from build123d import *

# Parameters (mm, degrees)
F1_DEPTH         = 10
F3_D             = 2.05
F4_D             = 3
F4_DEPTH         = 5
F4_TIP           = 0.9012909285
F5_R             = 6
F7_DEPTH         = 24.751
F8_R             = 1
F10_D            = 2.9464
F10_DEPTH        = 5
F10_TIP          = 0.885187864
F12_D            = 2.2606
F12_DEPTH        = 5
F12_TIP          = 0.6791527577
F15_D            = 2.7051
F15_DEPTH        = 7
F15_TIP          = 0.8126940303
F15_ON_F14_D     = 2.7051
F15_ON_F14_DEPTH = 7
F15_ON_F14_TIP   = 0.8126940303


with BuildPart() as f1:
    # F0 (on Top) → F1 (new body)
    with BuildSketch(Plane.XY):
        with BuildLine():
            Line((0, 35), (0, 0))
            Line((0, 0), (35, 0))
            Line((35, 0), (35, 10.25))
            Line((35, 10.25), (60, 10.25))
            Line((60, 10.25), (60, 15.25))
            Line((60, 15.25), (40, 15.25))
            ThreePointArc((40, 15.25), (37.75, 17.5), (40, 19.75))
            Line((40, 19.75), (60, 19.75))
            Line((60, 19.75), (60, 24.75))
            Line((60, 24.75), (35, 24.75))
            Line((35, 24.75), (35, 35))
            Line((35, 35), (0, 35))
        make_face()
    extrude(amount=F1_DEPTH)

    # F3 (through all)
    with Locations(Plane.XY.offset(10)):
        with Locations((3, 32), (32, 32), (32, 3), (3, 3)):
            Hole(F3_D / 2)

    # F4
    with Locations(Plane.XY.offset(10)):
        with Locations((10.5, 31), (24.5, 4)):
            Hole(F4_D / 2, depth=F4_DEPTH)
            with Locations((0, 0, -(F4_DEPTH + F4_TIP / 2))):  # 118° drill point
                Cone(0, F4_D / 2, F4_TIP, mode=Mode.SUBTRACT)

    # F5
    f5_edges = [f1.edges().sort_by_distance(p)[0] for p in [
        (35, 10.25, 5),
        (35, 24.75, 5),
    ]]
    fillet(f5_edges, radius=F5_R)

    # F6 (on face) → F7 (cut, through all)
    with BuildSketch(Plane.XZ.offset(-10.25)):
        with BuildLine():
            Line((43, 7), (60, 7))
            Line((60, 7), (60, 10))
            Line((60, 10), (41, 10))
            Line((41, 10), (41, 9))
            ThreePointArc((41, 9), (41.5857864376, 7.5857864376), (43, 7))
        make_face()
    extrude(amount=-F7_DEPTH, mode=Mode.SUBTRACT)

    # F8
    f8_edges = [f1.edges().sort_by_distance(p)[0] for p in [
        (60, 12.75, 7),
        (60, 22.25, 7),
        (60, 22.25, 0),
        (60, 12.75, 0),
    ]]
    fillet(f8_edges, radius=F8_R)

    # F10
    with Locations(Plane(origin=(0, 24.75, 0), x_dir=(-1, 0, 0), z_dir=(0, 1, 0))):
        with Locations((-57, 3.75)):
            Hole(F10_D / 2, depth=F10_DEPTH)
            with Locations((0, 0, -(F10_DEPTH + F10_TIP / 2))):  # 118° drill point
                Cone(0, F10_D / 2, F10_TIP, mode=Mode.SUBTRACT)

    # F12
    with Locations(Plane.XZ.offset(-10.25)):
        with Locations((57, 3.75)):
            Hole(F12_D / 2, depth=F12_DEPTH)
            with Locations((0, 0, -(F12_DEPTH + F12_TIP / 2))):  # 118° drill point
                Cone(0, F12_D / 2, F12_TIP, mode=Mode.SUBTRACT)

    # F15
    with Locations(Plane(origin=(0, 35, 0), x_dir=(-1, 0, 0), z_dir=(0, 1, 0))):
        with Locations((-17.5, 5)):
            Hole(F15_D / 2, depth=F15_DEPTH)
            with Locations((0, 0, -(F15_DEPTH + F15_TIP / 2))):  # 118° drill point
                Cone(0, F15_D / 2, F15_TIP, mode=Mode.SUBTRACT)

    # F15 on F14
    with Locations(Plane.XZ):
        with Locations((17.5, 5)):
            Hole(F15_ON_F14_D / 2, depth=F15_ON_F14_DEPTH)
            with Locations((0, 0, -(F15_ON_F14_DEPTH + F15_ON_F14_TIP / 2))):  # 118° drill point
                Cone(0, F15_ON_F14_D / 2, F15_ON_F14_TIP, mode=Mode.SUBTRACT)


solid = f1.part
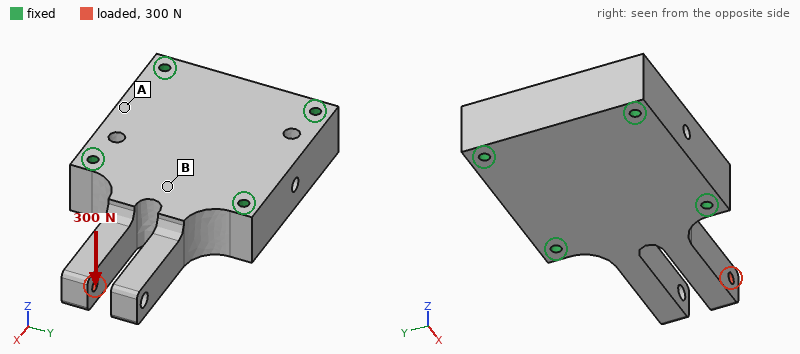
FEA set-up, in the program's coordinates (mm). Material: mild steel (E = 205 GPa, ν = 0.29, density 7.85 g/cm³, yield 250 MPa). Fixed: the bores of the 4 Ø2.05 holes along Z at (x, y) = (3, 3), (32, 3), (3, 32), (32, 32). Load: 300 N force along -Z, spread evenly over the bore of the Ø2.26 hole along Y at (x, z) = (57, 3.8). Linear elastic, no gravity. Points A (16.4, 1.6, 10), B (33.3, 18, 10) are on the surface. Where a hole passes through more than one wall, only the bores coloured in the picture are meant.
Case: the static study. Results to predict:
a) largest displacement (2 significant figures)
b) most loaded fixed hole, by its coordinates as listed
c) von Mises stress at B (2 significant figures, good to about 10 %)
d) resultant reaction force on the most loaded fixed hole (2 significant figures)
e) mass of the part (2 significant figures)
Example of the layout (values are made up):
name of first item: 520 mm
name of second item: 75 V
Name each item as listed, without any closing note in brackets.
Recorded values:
largest displacement: 38 µm
most loaded fixed hole, by its coordinates as listed: (32, 3)
von Mises stress at B: 24 MPa
resultant reaction force on the most loaded fixed hole: 330 N
mass of the part: 110 g
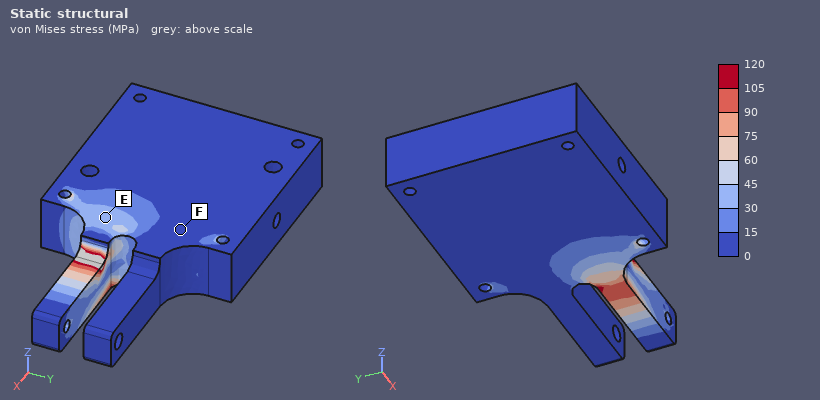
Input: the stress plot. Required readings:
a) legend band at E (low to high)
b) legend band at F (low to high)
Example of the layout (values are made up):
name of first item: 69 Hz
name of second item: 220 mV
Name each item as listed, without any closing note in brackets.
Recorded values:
legend band at E: 30 to 45 MPa
legend band at F: 0 to 15 MPa
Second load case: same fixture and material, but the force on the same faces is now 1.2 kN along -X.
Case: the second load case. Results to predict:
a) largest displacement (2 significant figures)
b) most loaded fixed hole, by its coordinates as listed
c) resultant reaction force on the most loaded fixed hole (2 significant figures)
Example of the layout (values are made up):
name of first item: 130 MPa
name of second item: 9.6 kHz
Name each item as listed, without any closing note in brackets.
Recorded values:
largest displacement: 5.1 µm
most loaded fixed hole, by its coordinates as listed: (32, 3)
resultant reaction force on the most loaded fixed hole: 530 N
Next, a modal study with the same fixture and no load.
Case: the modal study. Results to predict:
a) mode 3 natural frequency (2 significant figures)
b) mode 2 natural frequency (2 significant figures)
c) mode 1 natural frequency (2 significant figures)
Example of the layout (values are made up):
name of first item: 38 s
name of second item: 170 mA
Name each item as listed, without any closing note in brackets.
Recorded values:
mode 3 natural frequency: 9400 Hz
mode 2 natural frequency: 8600 Hz
mode 1 natural frequency: 8400 Hz
